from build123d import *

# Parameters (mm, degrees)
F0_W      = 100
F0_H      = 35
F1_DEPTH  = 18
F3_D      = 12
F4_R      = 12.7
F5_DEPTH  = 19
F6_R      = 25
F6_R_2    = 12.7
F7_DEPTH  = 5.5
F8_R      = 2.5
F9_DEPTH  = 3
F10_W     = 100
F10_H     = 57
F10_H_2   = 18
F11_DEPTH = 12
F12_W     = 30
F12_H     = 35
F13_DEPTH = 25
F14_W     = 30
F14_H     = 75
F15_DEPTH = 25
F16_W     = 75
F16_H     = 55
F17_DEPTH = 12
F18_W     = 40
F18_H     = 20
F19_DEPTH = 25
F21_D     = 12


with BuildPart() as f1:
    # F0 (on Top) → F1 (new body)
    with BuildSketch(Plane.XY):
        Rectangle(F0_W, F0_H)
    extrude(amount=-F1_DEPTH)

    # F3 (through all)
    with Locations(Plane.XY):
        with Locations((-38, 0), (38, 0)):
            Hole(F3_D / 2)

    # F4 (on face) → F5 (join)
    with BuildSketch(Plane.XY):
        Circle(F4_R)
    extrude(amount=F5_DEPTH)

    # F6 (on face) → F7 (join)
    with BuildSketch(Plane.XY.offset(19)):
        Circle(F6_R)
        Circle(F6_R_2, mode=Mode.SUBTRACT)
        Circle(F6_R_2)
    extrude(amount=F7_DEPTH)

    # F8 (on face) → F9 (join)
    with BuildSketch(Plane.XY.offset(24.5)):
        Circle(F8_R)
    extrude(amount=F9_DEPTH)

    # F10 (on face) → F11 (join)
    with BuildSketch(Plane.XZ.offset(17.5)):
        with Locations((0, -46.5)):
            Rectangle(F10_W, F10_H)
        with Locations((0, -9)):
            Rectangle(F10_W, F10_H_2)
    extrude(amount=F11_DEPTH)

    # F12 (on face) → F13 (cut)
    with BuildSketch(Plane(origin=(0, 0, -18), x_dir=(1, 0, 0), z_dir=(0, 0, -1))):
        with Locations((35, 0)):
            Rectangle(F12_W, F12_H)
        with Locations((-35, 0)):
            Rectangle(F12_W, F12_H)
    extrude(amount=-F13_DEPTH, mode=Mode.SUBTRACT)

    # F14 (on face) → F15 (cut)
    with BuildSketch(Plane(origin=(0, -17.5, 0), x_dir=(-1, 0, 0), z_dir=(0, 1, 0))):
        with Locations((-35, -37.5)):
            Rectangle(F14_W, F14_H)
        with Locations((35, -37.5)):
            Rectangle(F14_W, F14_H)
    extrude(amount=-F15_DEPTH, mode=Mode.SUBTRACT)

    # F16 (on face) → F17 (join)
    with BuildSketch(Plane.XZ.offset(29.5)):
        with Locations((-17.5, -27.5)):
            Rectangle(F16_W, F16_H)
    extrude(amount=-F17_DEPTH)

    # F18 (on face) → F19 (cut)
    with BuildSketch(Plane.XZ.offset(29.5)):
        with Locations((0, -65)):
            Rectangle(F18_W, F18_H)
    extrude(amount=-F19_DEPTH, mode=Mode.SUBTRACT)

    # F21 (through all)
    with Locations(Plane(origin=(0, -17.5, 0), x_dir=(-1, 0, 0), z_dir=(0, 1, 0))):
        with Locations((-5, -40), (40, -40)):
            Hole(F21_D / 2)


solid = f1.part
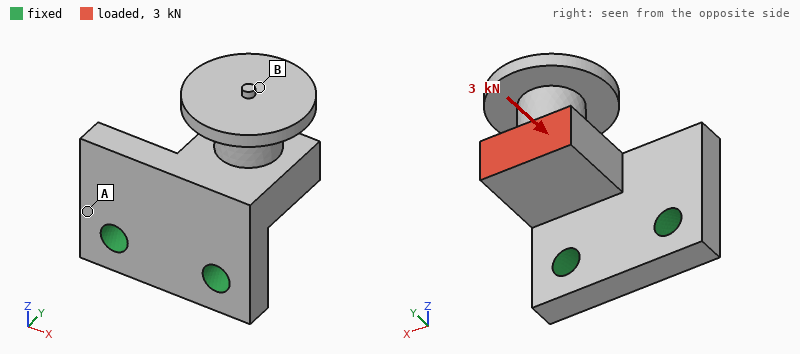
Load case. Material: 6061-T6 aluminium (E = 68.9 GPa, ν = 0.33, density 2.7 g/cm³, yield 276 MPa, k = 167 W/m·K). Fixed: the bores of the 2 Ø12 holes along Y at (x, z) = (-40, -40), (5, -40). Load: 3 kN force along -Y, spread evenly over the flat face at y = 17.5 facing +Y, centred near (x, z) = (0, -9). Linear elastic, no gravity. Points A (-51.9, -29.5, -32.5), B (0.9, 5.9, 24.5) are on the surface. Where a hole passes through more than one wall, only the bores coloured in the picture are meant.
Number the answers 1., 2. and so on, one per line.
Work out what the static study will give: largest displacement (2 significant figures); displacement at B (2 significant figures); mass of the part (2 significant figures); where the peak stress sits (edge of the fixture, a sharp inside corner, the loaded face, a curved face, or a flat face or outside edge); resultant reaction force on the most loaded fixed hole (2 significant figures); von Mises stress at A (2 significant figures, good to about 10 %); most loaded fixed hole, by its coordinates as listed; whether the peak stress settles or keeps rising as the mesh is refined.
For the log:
1. 0.15 mm
2. 0.13 mm
3. 250 g
4. edge of the fixture
5. 2.5 kN
6. 16 MPa
7. (5, -40)
8. keeps rising
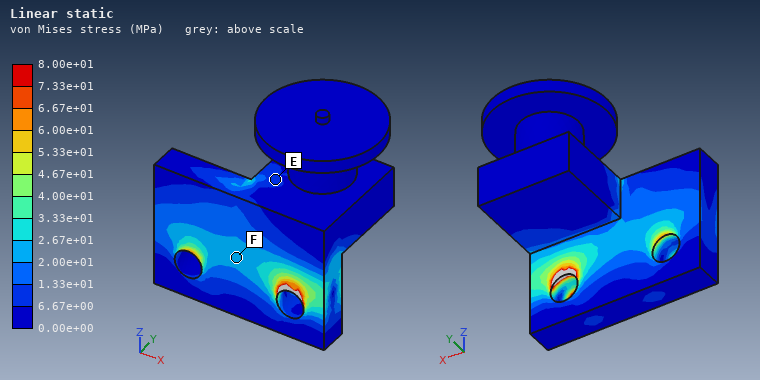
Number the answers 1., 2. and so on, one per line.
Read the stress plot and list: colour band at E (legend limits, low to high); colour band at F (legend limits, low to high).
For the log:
1. 6.67e+00 to 1.33e+01 MPa
2. 2.00e+01 to 2.67e+01 MPa
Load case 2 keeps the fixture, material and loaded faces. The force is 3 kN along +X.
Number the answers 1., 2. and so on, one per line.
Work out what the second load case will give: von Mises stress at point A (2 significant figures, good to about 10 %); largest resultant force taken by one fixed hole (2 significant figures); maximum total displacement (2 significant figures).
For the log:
1. 22 MPa
2. 3.2 kN
3. 0.11 mm
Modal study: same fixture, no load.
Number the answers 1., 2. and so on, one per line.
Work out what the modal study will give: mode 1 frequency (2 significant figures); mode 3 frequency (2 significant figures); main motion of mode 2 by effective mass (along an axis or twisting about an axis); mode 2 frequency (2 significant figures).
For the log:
1. 1600 Hz
2. 5800 Hz
3. along X
4. 3600 Hz
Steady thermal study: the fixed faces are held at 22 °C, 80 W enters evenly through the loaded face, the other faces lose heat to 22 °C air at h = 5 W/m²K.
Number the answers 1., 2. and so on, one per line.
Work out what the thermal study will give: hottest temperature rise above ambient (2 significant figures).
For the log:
1. 42 K
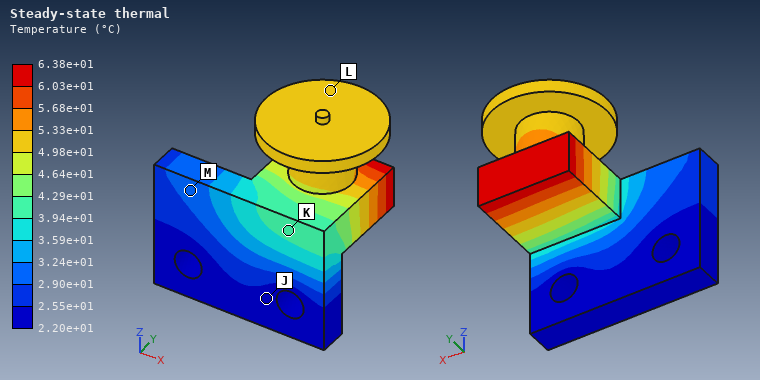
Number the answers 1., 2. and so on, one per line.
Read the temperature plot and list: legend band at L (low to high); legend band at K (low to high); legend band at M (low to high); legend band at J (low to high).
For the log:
1. 4.98e+01 to 5.33e+01 °C
2. 3.94e+01 to 4.29e+01 °C
3. 2.90e+01 to 3.24e+01 °C
4. 2.20e+01 to 2.55e+01 °C
